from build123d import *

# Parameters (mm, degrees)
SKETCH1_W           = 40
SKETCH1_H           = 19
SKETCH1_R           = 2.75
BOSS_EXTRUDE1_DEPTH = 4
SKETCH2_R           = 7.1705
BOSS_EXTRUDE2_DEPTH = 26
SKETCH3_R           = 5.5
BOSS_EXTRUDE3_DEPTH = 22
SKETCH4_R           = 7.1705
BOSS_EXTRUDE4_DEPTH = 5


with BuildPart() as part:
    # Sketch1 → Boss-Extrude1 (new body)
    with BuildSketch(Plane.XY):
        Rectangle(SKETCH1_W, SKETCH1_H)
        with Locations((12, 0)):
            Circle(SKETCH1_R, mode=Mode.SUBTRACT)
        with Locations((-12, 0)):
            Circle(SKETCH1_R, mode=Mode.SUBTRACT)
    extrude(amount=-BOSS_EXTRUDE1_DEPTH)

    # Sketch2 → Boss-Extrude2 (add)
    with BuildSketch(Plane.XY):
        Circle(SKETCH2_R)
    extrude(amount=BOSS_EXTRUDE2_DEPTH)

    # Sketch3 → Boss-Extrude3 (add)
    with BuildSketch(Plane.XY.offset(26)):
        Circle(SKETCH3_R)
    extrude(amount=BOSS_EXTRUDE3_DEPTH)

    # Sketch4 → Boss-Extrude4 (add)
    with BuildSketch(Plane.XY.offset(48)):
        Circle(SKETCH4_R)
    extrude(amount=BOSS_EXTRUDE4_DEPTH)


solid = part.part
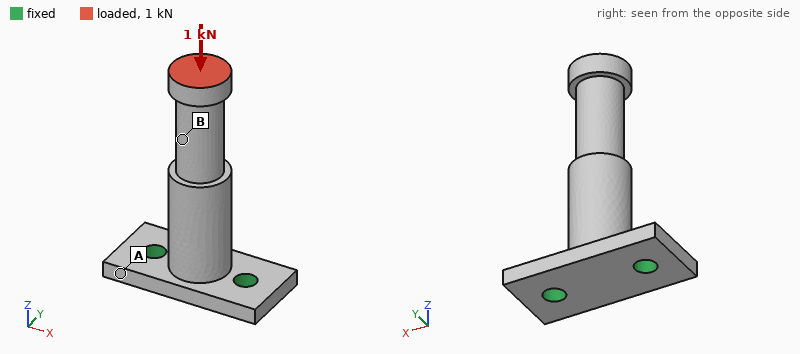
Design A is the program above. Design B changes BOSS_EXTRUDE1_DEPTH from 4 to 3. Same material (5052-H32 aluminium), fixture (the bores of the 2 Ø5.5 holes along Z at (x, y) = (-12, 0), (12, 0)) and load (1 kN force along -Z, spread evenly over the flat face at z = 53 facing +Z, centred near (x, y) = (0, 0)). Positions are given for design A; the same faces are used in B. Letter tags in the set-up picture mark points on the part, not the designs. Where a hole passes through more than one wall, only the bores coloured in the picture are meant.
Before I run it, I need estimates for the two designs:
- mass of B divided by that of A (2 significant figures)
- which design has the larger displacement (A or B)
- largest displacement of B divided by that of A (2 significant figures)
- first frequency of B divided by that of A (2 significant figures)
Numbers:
0.93
B
1.2
0.79
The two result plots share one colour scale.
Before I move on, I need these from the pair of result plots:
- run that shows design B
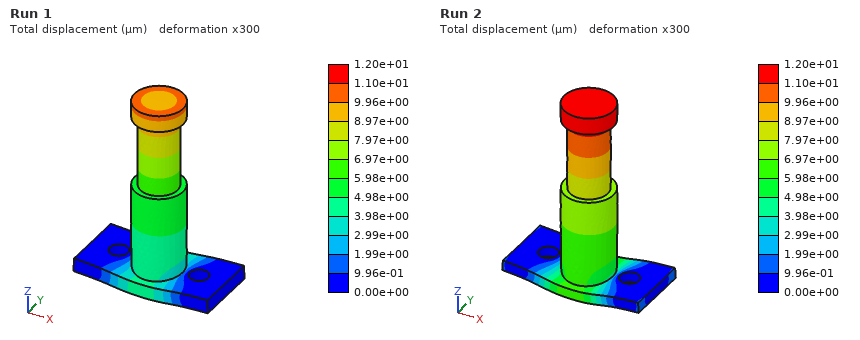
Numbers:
Run 2
